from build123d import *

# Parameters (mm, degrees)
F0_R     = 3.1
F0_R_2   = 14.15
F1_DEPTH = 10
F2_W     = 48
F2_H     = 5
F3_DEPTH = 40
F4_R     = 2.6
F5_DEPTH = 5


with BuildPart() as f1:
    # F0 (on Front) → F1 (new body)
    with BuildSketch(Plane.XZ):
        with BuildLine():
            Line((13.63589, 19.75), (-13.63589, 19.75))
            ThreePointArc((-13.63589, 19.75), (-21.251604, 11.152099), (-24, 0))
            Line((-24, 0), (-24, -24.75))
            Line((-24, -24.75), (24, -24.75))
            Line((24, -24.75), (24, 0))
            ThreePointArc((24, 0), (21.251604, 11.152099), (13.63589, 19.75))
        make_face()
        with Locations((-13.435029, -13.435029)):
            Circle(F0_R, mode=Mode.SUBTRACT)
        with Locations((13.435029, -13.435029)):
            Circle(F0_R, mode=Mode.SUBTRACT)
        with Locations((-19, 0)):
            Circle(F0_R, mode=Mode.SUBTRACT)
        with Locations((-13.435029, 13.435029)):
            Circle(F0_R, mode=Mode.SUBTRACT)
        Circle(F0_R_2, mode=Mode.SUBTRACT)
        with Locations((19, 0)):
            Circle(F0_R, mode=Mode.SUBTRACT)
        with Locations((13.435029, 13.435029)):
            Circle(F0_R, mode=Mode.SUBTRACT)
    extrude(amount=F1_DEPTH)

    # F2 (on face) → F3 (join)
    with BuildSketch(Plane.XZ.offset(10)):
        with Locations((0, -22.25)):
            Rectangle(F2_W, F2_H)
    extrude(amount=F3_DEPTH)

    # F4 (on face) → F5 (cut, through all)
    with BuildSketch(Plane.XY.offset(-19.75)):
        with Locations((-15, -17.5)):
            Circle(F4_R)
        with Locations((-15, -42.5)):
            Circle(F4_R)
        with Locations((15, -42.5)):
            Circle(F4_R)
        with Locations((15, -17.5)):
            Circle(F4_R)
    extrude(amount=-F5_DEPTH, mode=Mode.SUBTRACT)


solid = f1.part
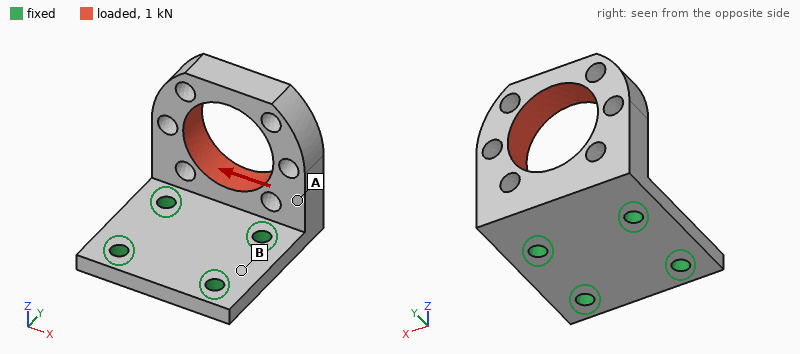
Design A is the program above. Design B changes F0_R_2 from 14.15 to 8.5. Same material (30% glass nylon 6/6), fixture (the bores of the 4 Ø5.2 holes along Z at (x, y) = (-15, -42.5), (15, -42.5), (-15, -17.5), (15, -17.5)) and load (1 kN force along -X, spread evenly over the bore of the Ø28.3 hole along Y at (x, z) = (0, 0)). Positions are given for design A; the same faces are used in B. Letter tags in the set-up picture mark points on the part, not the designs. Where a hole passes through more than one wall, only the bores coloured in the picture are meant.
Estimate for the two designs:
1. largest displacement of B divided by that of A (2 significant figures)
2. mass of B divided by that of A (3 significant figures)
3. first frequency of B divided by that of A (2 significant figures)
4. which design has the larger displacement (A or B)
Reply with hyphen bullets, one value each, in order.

- 0.63
- 1.19
- 0.90
- A
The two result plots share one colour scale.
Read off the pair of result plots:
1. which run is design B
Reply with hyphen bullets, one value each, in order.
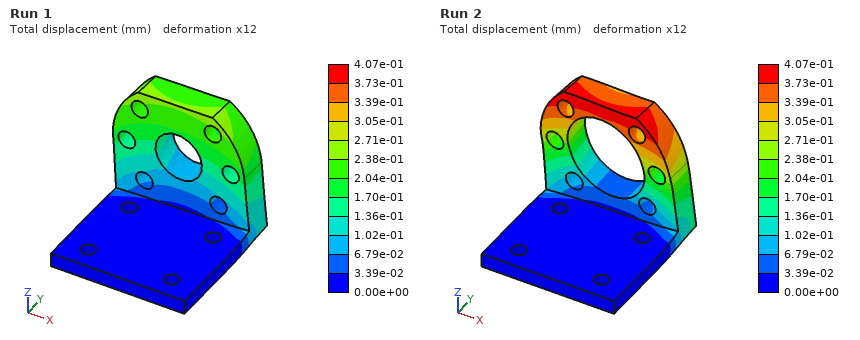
- Run 1
